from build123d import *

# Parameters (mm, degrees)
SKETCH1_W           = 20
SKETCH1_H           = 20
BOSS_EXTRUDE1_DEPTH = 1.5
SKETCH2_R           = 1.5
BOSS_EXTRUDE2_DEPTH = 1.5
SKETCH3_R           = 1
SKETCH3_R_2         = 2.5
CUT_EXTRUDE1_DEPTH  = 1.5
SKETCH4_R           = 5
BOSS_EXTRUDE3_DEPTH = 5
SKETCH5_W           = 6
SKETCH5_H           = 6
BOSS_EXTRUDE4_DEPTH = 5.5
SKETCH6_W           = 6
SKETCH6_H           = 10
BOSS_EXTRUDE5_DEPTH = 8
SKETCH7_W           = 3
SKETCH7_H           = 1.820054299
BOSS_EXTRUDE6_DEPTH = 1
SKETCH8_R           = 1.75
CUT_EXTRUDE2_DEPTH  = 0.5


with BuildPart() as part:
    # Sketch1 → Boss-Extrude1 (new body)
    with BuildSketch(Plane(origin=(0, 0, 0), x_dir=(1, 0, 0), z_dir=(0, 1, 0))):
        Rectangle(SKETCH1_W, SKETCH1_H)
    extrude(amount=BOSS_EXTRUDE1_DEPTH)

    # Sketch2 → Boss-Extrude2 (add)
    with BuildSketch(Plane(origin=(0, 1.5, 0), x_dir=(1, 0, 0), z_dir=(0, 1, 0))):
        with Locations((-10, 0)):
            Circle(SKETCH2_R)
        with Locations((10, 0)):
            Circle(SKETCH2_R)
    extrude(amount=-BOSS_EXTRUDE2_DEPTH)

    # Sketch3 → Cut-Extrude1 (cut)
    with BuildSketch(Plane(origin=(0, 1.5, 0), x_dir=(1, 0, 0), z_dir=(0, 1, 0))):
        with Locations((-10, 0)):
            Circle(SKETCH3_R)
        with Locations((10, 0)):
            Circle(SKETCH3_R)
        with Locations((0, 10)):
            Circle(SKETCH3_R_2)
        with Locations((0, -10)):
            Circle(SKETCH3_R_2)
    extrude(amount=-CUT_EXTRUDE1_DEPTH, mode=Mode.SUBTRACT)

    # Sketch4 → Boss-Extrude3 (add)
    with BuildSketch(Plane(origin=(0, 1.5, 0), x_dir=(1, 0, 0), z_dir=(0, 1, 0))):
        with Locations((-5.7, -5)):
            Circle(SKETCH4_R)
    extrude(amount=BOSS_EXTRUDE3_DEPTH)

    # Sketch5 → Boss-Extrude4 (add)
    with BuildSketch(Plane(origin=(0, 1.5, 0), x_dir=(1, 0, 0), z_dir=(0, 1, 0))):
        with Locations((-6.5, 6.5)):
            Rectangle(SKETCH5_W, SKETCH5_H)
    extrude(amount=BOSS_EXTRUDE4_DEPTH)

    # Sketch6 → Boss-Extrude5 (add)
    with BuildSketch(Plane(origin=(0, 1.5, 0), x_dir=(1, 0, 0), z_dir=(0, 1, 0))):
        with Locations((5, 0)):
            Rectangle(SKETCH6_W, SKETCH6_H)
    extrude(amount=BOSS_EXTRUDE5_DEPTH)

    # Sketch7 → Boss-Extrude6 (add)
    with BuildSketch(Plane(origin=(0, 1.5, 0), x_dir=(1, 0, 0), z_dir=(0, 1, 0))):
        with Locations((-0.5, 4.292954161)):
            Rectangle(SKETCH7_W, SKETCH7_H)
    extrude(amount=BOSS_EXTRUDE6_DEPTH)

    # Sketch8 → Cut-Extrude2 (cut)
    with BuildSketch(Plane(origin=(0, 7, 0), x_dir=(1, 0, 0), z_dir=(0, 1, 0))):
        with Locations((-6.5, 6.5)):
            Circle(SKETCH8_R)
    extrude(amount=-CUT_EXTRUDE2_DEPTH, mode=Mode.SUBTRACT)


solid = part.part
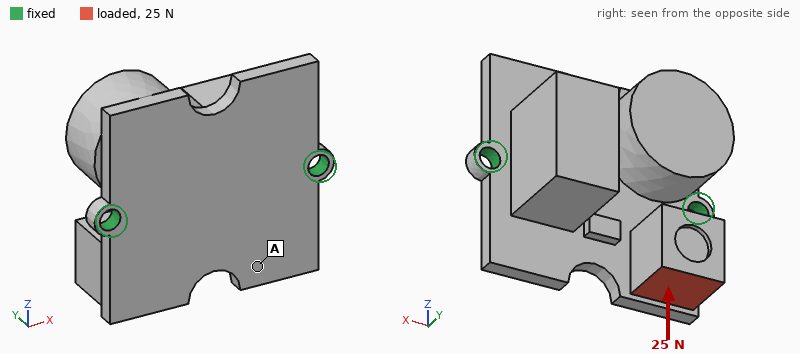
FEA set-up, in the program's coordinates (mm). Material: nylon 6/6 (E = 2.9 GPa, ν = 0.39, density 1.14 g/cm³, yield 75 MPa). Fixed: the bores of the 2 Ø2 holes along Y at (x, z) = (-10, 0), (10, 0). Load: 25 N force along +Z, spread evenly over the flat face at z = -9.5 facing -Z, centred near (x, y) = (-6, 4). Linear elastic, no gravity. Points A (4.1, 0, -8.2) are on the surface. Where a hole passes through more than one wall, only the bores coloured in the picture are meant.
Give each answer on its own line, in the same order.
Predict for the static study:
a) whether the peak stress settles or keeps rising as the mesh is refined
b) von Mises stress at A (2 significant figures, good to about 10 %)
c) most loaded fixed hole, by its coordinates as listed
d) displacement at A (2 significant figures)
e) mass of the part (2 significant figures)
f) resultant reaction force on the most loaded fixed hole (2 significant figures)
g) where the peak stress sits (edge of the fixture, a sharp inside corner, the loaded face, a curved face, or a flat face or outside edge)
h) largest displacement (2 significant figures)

keeps rising
2.9 MPa
(-10, 0)
0.093 mm
1.9 g
21 N
edge of the fixture
0.34 mm
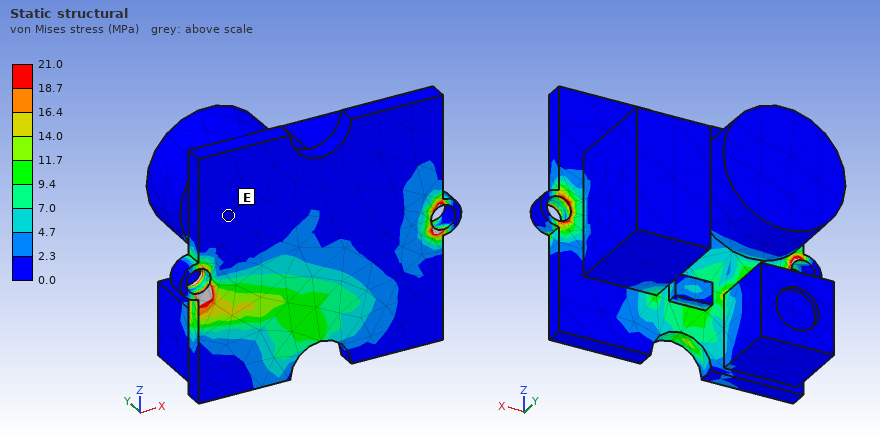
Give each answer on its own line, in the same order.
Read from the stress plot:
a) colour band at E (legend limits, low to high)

0.0 to 2.3 MPa
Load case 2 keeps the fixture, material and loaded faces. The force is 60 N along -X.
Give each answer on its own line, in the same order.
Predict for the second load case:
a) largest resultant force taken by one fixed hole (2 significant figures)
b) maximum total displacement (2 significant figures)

46 N
0.30 mm
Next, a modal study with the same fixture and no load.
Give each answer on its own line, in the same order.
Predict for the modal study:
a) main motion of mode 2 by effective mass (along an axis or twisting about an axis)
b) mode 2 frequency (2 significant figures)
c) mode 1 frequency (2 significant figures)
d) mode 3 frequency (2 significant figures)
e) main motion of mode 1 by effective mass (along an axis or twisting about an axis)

along Y
2500 Hz
1800 Hz
3400 Hz
along Z
